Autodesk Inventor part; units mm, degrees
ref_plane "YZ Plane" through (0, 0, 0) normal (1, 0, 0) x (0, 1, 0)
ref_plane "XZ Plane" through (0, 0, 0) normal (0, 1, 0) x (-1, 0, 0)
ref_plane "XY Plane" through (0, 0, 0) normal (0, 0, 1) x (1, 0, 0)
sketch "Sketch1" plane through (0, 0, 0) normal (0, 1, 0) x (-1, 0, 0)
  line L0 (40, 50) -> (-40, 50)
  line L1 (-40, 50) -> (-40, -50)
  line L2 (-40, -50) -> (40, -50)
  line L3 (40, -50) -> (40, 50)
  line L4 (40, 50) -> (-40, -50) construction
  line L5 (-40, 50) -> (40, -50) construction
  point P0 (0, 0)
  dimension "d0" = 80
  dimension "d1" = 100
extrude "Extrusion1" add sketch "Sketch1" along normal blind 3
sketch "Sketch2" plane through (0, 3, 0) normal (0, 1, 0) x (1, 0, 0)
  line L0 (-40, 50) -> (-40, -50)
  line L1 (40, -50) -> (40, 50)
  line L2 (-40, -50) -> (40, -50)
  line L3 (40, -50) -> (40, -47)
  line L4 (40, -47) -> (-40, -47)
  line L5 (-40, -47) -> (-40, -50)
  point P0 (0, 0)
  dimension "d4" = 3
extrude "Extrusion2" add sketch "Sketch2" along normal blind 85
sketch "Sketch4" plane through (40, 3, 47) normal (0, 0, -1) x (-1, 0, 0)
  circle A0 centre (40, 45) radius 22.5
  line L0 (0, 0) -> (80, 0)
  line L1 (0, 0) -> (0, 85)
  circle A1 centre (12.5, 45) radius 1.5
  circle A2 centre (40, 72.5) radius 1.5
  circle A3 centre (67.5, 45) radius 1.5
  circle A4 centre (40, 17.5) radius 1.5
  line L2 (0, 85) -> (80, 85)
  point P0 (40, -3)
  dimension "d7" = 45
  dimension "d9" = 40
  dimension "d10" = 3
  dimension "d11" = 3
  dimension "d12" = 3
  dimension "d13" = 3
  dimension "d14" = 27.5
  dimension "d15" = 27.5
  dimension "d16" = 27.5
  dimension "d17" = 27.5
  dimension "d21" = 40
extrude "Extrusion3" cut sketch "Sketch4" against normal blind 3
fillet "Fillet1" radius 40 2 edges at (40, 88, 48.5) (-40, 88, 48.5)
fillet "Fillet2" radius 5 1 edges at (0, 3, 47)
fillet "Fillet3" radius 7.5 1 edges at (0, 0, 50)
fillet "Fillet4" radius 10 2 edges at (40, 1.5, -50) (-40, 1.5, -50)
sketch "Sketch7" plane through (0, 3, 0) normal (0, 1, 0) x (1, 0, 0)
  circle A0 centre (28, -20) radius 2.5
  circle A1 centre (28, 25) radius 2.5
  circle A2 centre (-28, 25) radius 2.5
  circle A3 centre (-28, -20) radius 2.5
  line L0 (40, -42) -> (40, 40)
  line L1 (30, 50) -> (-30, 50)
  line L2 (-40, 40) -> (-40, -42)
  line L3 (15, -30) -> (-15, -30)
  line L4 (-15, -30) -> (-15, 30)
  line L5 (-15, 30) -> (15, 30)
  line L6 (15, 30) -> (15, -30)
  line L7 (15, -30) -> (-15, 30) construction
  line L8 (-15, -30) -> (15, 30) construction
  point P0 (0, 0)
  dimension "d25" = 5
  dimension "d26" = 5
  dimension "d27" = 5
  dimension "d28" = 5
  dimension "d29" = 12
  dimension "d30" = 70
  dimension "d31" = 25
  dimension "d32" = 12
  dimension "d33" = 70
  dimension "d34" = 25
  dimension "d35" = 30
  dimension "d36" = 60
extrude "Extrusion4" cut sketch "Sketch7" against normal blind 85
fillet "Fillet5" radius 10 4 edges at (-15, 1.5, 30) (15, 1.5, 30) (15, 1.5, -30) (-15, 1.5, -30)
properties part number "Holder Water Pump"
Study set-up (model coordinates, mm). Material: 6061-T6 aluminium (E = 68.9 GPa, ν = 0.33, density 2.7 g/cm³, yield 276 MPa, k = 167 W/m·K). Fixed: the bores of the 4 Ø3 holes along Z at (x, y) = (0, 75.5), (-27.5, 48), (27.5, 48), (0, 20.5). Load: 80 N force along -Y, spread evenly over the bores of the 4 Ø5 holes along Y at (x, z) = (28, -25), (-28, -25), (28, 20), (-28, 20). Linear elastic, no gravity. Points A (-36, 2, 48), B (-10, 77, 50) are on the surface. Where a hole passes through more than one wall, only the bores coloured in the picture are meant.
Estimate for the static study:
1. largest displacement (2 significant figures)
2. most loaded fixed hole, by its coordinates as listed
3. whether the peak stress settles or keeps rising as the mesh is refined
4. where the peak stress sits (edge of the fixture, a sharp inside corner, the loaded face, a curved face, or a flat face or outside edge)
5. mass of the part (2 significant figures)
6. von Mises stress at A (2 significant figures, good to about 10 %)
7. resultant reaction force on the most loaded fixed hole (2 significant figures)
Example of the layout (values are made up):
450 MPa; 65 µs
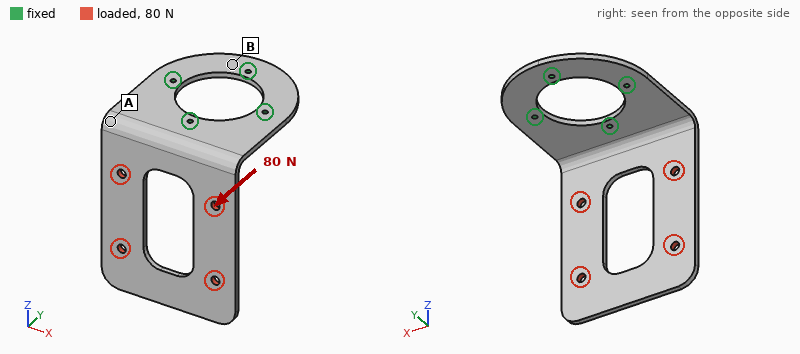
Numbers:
1.6 mm; (0, 20.5); keeps rising; edge of the fixture; 85 g; 26 MPa; 98 N
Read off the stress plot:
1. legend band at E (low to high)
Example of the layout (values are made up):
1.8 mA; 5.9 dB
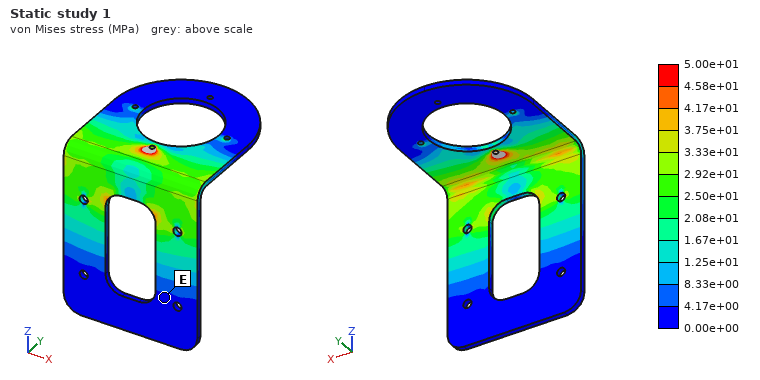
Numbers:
0.00e+00 to 4.17e+00 MPa
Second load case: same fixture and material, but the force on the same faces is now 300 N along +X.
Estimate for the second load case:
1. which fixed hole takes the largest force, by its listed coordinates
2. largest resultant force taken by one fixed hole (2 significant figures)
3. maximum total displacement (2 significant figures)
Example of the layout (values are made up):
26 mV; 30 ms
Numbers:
(0, 20.5); 240 N; 1.8 mm
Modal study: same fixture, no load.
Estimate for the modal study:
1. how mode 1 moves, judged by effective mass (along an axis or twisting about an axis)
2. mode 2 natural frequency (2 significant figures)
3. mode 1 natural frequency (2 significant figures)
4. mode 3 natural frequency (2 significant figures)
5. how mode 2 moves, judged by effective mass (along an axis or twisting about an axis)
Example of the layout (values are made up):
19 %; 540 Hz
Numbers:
along Y; 330 Hz; 190 Hz; 610 Hz; along X
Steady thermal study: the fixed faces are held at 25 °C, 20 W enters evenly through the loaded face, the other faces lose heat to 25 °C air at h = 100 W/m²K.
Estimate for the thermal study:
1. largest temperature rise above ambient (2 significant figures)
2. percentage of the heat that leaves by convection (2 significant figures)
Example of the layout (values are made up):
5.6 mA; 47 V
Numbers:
16 K; 77 %
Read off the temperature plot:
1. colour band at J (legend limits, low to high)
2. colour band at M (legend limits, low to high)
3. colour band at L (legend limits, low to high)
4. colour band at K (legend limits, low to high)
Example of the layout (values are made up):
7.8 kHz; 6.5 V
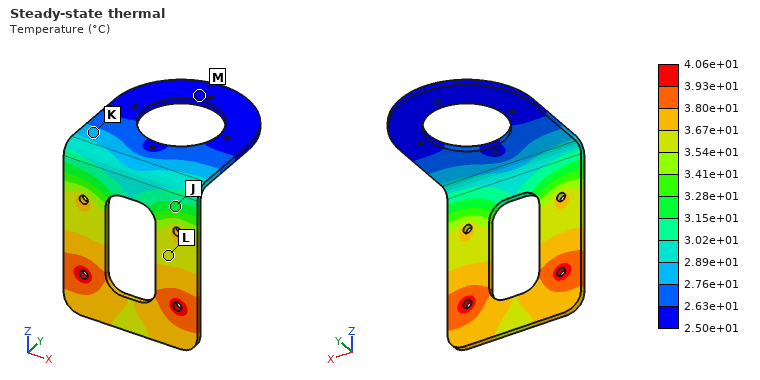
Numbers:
3.15e+01 to 3.28e+01 °C; 2.50e+01 to 2.63e+01 °C; 3.54e+01 to 3.67e+01 °C; 2.76e+01 to 2.89e+01 °C
